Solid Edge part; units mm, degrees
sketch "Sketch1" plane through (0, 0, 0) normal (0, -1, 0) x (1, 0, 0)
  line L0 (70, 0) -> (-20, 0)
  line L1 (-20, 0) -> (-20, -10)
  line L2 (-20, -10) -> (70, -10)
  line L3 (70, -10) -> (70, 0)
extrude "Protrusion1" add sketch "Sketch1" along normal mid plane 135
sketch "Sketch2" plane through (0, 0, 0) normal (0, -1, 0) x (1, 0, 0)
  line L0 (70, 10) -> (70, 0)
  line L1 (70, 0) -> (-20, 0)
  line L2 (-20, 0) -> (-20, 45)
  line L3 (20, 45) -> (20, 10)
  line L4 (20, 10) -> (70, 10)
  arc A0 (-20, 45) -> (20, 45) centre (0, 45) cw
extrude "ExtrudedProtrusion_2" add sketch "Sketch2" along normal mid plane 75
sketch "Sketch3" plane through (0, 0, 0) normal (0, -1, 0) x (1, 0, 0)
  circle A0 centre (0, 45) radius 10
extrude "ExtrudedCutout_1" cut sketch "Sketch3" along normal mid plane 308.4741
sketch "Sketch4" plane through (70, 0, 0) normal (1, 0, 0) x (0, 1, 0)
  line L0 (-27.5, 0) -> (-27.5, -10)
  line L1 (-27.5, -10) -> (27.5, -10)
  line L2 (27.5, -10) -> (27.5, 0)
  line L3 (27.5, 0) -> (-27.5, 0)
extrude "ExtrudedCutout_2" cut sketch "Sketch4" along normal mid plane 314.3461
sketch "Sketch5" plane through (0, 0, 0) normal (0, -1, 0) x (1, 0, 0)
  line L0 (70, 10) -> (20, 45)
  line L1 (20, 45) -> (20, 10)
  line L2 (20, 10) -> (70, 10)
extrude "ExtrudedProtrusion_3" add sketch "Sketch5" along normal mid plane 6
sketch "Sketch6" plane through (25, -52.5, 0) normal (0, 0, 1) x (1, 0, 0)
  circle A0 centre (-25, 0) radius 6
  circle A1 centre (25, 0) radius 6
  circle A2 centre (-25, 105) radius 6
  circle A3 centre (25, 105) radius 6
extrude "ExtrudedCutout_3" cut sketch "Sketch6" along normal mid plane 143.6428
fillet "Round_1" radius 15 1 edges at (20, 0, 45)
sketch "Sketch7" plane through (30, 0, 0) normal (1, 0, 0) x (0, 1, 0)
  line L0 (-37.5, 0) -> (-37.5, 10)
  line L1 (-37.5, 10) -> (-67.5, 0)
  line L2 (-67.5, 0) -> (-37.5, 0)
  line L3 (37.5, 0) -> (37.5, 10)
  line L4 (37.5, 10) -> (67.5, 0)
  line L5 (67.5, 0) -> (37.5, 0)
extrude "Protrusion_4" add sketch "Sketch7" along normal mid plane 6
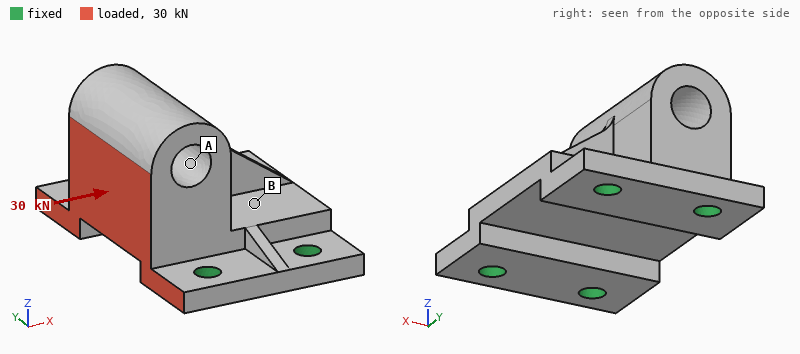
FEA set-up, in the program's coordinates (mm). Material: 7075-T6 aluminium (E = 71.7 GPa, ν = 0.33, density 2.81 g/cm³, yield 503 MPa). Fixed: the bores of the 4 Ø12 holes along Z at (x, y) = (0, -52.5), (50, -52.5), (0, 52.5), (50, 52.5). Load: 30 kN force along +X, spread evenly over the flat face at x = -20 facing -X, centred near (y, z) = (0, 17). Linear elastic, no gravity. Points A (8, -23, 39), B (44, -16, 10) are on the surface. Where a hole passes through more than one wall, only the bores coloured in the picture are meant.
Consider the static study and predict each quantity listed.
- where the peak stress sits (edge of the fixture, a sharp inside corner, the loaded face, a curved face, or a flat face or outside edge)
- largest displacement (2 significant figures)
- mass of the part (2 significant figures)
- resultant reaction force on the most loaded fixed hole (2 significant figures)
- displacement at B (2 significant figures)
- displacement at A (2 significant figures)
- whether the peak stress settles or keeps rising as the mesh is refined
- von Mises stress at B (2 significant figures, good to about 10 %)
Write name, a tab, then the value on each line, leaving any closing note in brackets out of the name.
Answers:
where the peak stress sits	edge of the fixture
largest displacement	0.17 mm
mass of the part	760 g
resultant reaction force on the most loaded fixed hole	13 kN
displacement at B	0.051 mm
displacement at A	0.11 mm
whether the peak stress settles or keeps rising as the mesh is refined	keeps rising
von Mises stress at B	34 MPa
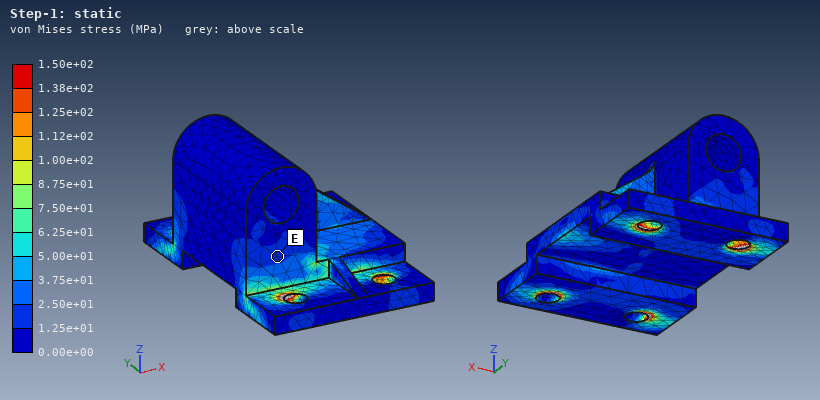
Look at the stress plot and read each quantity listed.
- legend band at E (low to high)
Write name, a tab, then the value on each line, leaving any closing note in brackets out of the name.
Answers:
legend band at E	1.25e+01 to 2.50e+01 MPa
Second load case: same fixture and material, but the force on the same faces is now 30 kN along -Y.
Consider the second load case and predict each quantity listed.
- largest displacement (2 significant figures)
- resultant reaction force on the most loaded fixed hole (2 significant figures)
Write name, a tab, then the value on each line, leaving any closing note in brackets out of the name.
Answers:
largest displacement	60 µm
resultant reaction force on the most loaded fixed hole	14 kN
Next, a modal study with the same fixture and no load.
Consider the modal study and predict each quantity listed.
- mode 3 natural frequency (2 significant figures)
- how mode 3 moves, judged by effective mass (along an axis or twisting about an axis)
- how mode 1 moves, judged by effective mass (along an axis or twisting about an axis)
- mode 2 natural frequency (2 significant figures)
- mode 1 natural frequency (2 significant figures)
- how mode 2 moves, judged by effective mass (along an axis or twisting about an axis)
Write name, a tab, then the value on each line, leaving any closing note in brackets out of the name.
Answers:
mode 3 natural frequency	5200 Hz
how mode 3 moves, judged by effective mass	along Z
how mode 1 moves, judged by effective mass	along X
mode 2 natural frequency	5000 Hz
mode 1 natural frequency	2900 Hz
how mode 2 moves, judged by effective mass	along Y
